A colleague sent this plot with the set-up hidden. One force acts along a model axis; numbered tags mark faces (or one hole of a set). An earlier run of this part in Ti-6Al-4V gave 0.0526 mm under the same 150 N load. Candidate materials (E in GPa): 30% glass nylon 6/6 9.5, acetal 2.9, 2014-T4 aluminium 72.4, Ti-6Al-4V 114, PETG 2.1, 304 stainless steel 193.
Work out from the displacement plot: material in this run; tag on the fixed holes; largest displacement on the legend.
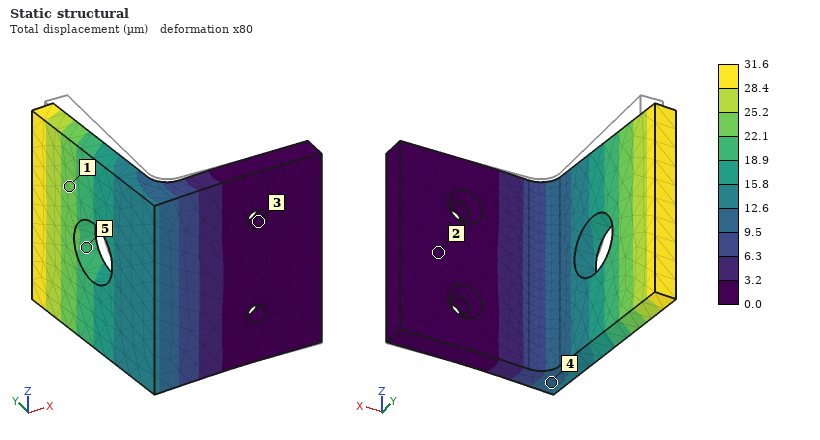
304 stainless steel
3
31.6 µm
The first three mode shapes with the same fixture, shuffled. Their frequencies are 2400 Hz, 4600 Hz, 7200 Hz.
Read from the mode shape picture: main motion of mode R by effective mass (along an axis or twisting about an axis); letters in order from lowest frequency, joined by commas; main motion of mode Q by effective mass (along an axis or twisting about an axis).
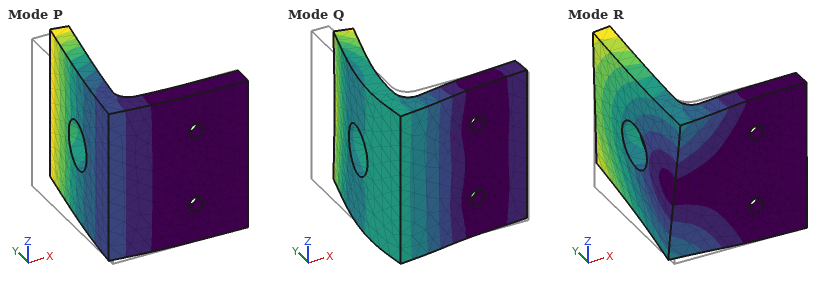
along Z
P, R, Q
along Y
